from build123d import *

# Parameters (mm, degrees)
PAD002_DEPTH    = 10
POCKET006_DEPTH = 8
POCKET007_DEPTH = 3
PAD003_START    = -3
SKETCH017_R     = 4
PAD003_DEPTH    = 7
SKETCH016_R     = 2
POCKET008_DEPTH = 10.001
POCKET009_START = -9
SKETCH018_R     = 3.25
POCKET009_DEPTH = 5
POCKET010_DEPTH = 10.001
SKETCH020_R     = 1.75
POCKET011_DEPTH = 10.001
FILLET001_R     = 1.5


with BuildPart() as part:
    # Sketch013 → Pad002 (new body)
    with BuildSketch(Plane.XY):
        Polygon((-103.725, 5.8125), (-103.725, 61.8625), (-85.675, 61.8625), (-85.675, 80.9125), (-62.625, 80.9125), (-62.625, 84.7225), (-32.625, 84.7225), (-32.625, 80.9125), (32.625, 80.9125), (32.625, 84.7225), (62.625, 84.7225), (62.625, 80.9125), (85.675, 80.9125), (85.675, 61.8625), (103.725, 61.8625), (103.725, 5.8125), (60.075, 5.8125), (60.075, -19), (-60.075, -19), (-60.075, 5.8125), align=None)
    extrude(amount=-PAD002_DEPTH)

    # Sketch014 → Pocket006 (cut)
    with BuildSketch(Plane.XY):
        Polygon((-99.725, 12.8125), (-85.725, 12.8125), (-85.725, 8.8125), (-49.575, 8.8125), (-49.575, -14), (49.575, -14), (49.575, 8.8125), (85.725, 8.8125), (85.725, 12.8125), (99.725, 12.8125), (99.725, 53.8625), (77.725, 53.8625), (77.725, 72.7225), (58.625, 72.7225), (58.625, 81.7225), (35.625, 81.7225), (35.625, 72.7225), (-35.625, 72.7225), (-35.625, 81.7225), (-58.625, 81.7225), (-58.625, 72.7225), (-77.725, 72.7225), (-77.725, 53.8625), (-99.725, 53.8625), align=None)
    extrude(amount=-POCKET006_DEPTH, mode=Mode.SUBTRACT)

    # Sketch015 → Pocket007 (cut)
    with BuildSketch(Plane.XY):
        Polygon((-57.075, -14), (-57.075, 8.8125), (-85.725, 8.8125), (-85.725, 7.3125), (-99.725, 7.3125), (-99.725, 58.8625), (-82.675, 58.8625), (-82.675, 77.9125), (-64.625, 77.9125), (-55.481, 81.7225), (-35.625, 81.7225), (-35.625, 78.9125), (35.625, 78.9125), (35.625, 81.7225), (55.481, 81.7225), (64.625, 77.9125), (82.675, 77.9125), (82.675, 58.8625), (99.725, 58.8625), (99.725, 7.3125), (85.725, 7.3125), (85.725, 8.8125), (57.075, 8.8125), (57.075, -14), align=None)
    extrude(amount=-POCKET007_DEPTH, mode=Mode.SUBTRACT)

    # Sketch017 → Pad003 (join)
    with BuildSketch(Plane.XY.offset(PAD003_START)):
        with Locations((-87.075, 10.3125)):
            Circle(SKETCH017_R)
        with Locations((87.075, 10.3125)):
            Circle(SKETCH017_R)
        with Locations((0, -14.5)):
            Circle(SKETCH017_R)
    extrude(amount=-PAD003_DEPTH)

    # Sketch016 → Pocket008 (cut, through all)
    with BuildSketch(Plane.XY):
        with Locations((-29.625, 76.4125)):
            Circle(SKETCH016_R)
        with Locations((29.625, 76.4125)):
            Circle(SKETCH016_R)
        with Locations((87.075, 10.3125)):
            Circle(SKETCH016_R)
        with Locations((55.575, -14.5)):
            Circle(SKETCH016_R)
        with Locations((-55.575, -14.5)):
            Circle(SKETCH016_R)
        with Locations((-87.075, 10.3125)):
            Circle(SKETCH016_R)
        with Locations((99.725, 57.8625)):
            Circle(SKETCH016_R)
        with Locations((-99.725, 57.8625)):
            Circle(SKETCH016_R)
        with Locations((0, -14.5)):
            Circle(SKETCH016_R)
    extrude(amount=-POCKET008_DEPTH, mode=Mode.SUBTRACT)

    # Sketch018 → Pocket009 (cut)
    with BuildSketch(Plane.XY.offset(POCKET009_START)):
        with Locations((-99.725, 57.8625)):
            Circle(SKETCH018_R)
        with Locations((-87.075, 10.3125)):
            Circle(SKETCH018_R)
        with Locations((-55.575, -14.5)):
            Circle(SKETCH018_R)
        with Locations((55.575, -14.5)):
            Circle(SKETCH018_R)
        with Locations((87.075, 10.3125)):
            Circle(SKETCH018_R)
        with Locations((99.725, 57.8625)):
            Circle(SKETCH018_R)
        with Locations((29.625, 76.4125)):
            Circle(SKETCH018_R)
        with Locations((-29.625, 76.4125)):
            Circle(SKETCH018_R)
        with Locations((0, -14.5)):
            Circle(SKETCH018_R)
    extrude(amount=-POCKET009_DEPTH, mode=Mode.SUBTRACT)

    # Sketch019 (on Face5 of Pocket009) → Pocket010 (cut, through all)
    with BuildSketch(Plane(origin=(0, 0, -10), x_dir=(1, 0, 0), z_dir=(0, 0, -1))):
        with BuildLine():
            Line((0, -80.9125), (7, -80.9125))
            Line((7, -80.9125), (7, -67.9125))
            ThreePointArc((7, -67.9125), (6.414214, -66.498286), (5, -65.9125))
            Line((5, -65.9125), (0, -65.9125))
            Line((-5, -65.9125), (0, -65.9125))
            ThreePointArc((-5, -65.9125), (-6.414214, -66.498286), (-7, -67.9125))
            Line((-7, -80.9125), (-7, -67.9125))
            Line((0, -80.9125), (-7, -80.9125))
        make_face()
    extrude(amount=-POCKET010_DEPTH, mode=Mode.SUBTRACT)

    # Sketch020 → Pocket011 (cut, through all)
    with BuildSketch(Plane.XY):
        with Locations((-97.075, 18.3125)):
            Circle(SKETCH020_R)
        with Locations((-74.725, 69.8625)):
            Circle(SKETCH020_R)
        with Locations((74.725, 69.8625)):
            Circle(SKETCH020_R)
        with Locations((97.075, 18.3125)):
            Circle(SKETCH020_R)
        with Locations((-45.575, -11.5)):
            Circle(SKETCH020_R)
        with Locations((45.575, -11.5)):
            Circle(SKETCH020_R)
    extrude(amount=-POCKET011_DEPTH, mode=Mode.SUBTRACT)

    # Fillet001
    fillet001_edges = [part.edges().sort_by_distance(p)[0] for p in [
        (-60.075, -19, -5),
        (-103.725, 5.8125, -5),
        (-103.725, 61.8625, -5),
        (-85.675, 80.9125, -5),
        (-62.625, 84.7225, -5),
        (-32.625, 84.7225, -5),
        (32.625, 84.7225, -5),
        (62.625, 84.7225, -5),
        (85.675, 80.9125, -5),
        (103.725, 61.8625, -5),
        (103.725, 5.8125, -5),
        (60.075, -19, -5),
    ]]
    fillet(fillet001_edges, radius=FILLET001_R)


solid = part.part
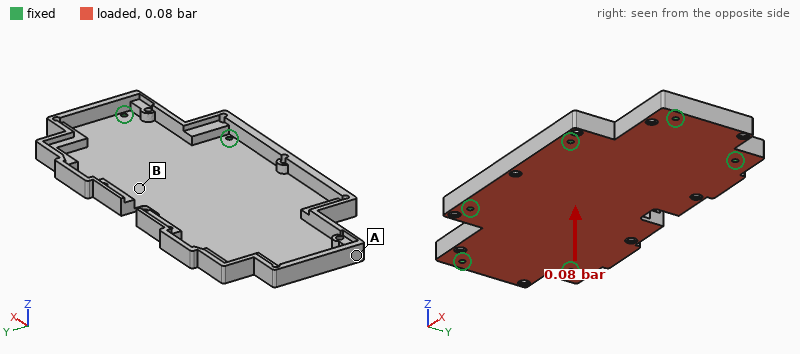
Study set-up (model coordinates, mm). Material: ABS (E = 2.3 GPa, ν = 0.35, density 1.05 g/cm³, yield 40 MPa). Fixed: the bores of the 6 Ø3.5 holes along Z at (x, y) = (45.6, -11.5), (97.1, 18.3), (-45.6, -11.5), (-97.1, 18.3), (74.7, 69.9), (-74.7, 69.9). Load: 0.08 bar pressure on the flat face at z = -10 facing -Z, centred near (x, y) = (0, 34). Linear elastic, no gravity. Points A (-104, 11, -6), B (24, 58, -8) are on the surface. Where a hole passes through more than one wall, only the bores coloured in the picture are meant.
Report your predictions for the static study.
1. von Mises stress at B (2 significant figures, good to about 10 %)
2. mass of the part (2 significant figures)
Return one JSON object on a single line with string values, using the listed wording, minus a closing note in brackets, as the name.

{"von Mises stress at B": "3.2 MPa", "mass of the part": "61 g"}
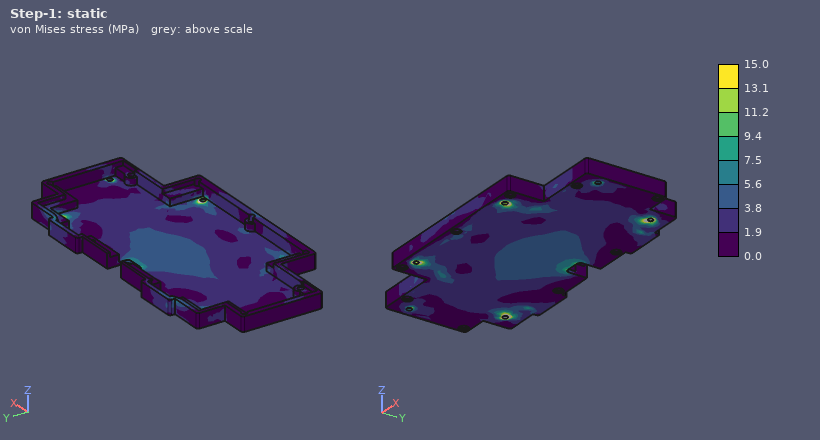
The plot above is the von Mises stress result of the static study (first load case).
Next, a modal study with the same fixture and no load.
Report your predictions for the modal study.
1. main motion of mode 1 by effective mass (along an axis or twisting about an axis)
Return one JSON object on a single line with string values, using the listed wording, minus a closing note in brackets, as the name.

{"main motion of mode 1 by effective mass": "along Z"}
